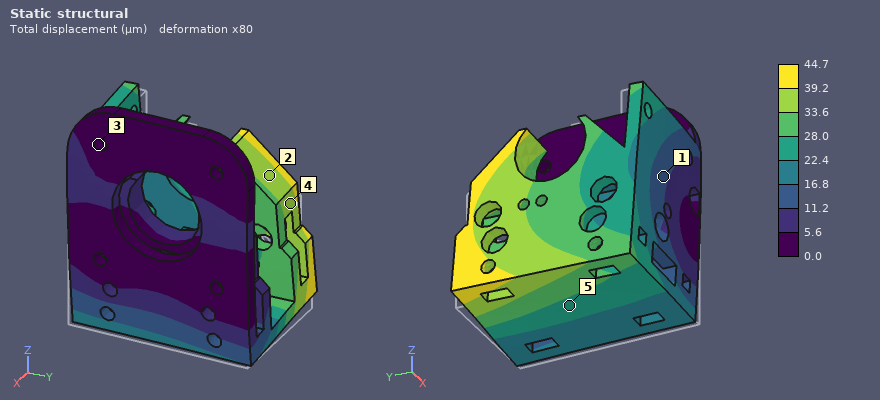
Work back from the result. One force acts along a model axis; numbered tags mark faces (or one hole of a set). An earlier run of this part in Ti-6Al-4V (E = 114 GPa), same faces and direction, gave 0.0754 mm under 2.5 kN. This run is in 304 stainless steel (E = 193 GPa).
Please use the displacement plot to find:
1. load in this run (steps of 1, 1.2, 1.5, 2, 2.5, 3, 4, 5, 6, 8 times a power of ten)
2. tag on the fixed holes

2.5 kN
3
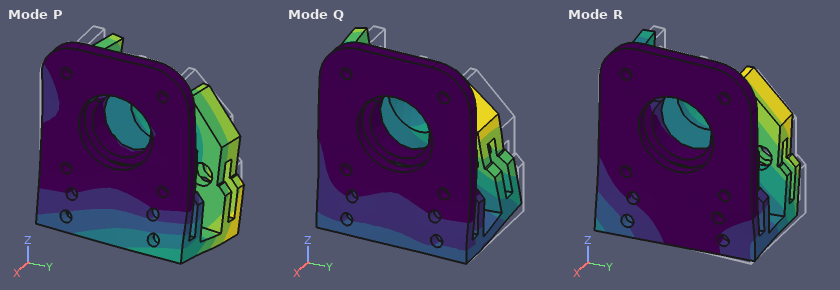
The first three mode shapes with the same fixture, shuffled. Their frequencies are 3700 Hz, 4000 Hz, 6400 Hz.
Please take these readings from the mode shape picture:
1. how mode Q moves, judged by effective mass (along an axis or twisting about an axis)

along X
